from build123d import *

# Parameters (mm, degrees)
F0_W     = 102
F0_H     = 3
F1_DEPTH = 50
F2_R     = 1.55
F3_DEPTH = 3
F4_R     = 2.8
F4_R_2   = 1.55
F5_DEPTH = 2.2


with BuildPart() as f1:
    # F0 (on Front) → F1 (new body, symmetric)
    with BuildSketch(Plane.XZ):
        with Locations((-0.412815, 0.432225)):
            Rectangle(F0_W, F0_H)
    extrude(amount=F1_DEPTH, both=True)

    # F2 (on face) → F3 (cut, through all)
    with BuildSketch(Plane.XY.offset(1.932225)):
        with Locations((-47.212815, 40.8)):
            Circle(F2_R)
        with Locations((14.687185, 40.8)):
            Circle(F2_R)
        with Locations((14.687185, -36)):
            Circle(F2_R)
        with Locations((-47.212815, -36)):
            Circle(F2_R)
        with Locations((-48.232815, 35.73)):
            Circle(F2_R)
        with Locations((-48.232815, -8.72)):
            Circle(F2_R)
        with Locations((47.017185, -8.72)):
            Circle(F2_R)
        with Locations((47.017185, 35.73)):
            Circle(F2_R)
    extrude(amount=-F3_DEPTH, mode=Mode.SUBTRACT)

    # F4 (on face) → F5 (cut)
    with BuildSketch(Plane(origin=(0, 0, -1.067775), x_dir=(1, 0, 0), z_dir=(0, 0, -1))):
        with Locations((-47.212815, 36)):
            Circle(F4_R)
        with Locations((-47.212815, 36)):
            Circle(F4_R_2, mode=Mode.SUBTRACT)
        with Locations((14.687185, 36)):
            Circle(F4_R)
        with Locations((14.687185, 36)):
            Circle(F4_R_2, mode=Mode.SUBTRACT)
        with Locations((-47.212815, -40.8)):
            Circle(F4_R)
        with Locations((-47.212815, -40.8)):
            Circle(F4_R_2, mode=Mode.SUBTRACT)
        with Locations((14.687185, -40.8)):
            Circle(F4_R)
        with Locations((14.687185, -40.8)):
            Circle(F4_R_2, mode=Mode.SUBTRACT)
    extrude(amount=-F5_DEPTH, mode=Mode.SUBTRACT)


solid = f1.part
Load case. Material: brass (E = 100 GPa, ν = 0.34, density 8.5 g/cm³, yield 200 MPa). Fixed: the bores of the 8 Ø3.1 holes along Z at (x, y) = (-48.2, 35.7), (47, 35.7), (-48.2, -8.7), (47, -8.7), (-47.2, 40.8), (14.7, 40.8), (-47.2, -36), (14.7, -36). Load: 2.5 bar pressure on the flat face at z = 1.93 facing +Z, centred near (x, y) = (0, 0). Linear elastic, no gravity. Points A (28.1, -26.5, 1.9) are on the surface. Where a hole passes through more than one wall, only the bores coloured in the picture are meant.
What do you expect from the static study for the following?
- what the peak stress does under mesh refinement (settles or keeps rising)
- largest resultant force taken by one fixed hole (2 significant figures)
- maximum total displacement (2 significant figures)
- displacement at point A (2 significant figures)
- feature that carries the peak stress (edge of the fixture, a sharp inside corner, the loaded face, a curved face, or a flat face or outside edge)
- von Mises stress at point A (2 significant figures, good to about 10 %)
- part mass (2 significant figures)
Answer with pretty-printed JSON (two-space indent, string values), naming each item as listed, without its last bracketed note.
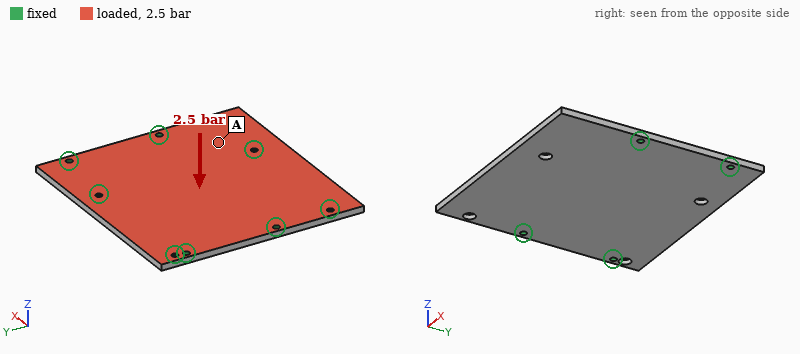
{
  "what the peak stress does under mesh refinement": "keeps rising",
  "largest resultant force taken by one fixed hole": "820 N",
  "maximum total displacement": "0.14 mm",
  "displacement at point A": "0.023 mm",
  "feature that carries the peak stress": "edge of the fixture",
  "von Mises stress at point A": "36 MPa",
  "part mass": "260 g"
}
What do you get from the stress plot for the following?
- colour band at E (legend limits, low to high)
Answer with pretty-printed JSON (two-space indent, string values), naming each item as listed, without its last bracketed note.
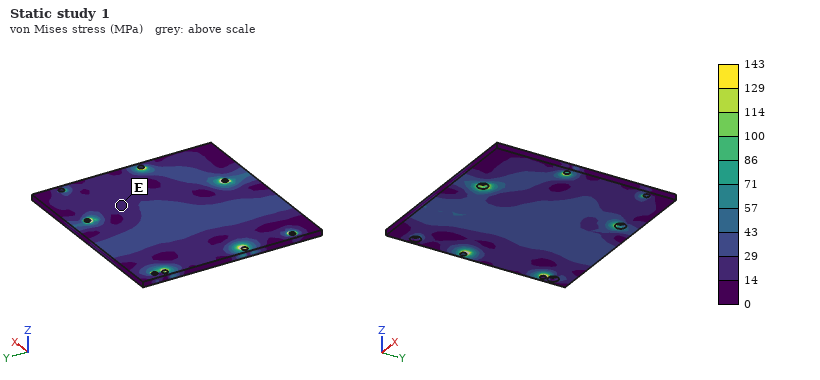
{
  "colour band at E": "14 to 29 MPa"
}
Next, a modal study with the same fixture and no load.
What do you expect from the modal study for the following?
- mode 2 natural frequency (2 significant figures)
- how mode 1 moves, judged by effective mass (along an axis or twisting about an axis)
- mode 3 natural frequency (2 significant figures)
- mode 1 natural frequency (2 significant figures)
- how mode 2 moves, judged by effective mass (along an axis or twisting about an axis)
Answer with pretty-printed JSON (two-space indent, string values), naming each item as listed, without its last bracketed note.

{
  "mode 2 natural frequency": "1900 Hz",
  "how mode 1 moves, judged by effective mass": "along Z",
  "mode 3 natural frequency": "2200 Hz",
  "mode 1 natural frequency": "1500 Hz",
  "how mode 2 moves, judged by effective mass": "along Z"
}
